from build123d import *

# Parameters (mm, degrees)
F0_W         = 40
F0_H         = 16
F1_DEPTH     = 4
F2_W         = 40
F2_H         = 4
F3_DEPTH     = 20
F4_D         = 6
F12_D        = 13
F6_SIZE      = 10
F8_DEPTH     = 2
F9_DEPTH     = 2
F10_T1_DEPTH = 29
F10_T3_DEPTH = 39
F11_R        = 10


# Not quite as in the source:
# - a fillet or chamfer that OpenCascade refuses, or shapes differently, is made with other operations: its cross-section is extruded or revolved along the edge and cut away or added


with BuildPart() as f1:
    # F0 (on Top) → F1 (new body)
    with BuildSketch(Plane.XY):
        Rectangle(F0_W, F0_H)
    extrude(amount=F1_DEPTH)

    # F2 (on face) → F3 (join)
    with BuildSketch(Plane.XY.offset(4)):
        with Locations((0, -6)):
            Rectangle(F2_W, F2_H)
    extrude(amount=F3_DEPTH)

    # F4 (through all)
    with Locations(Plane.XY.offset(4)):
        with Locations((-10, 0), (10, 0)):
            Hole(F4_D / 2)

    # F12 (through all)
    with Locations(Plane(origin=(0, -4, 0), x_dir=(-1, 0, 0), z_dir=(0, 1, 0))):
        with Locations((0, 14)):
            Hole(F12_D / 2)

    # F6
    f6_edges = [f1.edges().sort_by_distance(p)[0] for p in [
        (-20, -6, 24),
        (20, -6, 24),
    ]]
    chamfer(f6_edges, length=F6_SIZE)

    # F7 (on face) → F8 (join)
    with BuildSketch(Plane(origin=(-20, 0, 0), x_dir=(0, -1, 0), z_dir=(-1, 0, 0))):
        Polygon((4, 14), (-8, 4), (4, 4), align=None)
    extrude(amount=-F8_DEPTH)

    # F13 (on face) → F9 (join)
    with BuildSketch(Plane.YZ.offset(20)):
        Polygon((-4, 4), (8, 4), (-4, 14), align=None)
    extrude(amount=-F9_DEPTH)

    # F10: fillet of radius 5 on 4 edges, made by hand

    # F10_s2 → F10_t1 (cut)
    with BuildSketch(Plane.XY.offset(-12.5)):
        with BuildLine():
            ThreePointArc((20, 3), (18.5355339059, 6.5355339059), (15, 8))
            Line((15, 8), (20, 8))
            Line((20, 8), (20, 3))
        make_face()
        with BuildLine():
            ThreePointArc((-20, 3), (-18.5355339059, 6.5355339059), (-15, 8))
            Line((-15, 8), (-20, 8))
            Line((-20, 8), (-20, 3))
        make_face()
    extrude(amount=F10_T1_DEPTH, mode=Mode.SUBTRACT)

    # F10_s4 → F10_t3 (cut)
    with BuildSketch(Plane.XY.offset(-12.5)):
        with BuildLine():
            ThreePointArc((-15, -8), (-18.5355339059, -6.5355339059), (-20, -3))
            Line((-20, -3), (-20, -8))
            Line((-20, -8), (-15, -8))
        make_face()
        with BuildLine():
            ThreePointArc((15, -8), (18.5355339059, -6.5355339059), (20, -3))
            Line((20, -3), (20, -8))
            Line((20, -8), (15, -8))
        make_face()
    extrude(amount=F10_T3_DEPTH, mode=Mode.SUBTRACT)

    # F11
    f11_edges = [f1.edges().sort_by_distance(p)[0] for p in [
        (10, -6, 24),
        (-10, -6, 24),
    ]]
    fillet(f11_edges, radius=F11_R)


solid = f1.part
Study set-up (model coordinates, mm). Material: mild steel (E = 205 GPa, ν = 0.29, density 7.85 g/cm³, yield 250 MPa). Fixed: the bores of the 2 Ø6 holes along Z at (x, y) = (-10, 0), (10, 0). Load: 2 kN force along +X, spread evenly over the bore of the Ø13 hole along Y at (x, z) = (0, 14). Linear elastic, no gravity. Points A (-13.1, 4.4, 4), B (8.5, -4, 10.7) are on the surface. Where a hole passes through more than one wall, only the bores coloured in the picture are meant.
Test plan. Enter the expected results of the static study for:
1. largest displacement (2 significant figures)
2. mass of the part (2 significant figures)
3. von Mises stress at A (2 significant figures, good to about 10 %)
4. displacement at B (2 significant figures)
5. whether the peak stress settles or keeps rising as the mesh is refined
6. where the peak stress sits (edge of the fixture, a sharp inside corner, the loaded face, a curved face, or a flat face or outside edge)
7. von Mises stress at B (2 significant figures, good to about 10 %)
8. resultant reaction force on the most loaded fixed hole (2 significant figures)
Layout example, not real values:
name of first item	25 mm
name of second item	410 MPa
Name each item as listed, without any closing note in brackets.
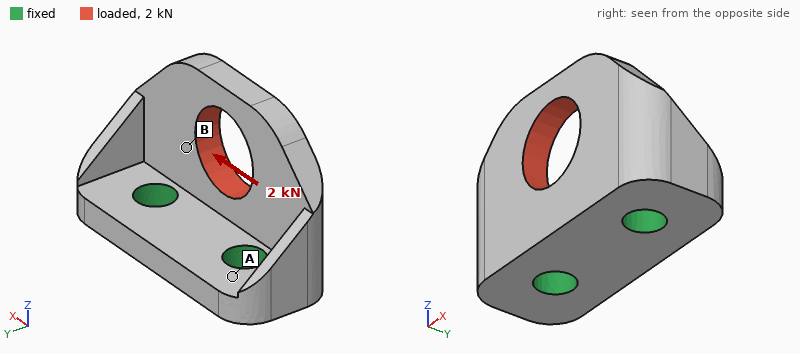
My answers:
largest displacement	14 µm
mass of the part	36 g
von Mises stress at A	18 MPa
displacement at B	5.8 µm
whether the peak stress settles or keeps rising as the mesh is refined	keeps rising
where the peak stress sits	edge of the fixture
von Mises stress at B	44 MPa
resultant reaction force on the most loaded fixed hole	1.4 kN
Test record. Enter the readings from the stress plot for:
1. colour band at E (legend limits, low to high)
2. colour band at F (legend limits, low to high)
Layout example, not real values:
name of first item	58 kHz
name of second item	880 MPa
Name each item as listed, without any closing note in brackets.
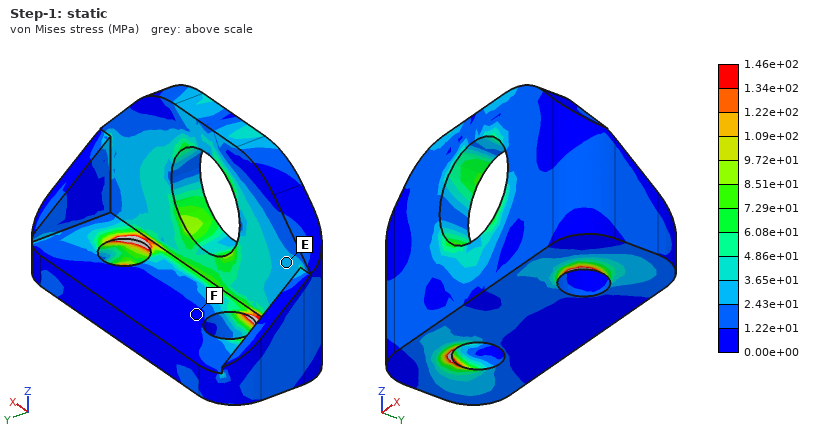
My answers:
colour band at E	2.43e+01 to 3.65e+01 MPa
colour band at F	0.00e+00 to 1.22e+01 MPa
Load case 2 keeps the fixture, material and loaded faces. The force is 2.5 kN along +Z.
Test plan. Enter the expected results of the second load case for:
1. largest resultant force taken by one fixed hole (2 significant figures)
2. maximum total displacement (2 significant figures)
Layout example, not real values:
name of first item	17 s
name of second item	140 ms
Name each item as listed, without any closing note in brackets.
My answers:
largest resultant force taken by one fixed hole	1.3 kN
maximum total displacement	16 µm
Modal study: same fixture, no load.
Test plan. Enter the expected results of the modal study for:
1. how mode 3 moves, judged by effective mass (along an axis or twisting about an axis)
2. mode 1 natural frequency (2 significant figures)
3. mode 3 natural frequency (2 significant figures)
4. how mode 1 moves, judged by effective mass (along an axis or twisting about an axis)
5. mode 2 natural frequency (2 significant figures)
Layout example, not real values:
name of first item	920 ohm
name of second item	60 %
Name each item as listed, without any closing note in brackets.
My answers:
how mode 3 moves, judged by effective mass	along X
mode 1 natural frequency	7500 Hz
mode 3 natural frequency	19 kHz
how mode 1 moves, judged by effective mass	along Y
mode 2 natural frequency	13 kHz
